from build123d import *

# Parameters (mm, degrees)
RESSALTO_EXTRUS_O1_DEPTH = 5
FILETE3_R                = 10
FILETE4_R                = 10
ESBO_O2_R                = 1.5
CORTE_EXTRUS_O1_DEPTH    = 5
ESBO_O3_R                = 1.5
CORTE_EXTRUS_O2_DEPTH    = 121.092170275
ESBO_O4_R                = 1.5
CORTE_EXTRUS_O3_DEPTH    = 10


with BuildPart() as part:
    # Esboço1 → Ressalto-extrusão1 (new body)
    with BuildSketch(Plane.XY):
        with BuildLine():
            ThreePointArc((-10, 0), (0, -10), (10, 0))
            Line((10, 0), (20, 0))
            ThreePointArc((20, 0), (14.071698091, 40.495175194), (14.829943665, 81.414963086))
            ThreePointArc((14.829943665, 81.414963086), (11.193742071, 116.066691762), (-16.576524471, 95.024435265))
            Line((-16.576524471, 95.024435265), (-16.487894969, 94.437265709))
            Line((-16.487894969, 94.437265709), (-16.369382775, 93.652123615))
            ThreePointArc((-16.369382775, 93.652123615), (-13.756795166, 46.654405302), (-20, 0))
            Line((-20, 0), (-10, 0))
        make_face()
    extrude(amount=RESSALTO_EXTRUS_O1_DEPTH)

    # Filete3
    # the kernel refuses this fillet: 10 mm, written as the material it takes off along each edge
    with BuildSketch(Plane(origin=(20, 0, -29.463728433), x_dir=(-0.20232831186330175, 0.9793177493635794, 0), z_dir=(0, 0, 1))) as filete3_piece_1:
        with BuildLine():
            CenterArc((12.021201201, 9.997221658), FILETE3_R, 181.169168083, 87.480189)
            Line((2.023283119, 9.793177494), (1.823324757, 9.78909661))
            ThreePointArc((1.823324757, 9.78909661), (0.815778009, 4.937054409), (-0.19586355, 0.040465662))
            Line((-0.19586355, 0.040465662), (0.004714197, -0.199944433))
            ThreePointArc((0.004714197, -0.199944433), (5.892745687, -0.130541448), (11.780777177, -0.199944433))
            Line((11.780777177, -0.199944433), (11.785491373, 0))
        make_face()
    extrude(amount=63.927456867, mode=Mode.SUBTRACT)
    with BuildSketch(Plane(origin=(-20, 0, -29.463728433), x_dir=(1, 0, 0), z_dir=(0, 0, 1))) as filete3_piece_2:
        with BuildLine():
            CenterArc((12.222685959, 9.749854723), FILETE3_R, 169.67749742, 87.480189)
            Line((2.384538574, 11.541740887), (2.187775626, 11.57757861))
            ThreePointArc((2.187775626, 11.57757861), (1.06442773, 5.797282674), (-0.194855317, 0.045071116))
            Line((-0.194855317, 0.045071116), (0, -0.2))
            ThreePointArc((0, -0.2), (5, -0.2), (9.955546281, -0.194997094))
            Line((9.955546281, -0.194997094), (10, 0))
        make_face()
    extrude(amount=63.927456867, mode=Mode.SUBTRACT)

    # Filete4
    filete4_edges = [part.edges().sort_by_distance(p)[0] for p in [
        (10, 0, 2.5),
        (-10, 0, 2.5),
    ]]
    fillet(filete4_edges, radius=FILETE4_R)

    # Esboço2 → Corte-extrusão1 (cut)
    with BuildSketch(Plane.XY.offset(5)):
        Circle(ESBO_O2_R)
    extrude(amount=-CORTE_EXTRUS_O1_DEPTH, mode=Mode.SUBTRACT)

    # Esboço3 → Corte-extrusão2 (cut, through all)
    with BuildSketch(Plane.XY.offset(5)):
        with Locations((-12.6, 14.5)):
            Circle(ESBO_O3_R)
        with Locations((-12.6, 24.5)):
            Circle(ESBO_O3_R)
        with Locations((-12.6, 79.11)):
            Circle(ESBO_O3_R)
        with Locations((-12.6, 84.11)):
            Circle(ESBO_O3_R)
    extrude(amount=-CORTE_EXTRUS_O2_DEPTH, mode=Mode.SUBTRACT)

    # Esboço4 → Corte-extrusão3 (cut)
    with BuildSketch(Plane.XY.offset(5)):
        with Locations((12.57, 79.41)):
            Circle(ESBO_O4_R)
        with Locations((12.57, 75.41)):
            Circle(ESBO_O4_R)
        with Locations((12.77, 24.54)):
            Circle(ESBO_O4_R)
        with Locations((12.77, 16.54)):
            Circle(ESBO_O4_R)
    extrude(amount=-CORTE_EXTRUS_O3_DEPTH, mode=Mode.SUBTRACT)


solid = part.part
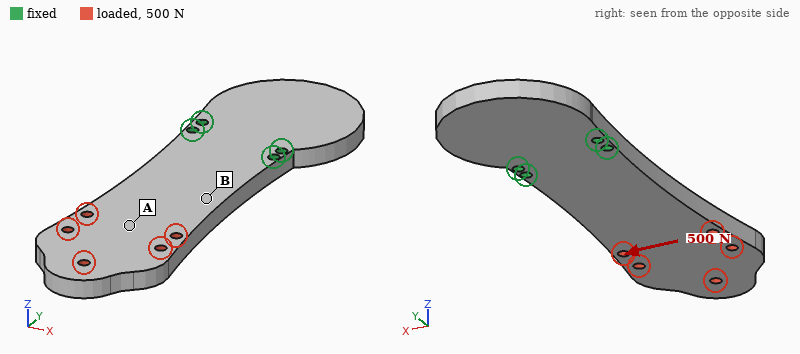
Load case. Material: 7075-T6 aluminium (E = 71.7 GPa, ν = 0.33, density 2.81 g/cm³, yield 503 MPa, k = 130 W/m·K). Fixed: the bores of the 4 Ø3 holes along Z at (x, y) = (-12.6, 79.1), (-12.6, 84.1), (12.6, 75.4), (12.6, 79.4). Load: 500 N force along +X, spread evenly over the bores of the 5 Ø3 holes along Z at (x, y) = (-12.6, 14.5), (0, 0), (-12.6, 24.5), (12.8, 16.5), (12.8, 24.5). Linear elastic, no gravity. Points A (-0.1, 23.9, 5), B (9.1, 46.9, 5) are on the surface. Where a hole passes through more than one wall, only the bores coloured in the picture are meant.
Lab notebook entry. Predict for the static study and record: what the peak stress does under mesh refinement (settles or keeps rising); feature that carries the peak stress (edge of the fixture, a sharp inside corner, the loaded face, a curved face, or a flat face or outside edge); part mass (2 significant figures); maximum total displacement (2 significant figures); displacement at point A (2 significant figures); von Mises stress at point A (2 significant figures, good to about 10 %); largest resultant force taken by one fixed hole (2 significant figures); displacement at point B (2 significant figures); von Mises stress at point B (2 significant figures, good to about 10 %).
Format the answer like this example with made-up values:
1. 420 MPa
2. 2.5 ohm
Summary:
1. keeps rising
2. edge of the fixture
3. 52 g
4. 0.11 mm
5. 0.055 mm
6. 7.1 MPa
7. 1.1 kN
8. 0.024 mm
9. 17 MPa
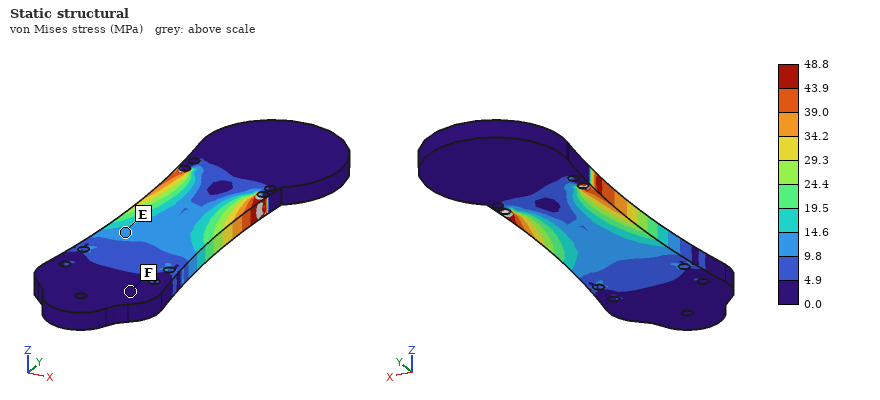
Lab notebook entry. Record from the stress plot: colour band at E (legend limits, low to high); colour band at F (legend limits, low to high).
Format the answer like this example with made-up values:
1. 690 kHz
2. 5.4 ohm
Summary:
1. 9.8 to 14.6 MPa
2. 0.0 to 4.9 MPa
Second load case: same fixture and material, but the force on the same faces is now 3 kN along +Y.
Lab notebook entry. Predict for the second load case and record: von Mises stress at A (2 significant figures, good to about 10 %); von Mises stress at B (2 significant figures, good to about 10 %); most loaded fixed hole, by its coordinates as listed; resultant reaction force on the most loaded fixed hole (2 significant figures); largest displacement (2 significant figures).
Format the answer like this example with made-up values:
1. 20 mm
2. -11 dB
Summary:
1. 14 MPa
2. 22 MPa
3. (-12.6, 79.1)
4. 1.1 kN
5. 21 µm
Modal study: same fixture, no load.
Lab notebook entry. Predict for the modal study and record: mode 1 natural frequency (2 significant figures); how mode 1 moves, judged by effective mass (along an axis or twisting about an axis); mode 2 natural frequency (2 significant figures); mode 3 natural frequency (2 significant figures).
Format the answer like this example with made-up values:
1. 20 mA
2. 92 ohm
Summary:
1. 550 Hz
2. along Z
3. 2900 Hz
4. 3000 Hz
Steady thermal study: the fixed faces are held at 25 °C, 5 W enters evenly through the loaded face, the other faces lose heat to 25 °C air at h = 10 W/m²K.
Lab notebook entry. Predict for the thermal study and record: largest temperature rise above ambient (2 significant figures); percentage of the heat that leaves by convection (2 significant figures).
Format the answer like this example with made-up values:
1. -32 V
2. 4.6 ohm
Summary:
1. 16 K
2. 12 %
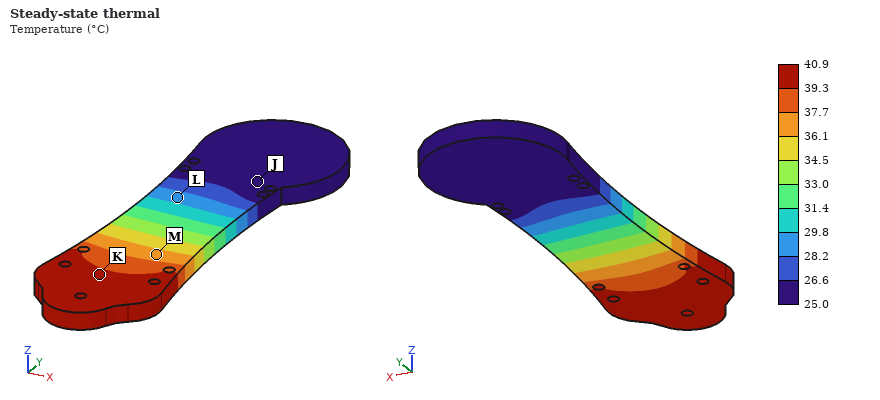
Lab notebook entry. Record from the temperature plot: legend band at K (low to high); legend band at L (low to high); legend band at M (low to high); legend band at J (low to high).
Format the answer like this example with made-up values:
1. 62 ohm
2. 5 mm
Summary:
1. 39.3 to 40.9 °C
2. 28.2 to 29.8 °C
3. 36.1 to 37.7 °C
4. 25.0 to 26.6 °C
